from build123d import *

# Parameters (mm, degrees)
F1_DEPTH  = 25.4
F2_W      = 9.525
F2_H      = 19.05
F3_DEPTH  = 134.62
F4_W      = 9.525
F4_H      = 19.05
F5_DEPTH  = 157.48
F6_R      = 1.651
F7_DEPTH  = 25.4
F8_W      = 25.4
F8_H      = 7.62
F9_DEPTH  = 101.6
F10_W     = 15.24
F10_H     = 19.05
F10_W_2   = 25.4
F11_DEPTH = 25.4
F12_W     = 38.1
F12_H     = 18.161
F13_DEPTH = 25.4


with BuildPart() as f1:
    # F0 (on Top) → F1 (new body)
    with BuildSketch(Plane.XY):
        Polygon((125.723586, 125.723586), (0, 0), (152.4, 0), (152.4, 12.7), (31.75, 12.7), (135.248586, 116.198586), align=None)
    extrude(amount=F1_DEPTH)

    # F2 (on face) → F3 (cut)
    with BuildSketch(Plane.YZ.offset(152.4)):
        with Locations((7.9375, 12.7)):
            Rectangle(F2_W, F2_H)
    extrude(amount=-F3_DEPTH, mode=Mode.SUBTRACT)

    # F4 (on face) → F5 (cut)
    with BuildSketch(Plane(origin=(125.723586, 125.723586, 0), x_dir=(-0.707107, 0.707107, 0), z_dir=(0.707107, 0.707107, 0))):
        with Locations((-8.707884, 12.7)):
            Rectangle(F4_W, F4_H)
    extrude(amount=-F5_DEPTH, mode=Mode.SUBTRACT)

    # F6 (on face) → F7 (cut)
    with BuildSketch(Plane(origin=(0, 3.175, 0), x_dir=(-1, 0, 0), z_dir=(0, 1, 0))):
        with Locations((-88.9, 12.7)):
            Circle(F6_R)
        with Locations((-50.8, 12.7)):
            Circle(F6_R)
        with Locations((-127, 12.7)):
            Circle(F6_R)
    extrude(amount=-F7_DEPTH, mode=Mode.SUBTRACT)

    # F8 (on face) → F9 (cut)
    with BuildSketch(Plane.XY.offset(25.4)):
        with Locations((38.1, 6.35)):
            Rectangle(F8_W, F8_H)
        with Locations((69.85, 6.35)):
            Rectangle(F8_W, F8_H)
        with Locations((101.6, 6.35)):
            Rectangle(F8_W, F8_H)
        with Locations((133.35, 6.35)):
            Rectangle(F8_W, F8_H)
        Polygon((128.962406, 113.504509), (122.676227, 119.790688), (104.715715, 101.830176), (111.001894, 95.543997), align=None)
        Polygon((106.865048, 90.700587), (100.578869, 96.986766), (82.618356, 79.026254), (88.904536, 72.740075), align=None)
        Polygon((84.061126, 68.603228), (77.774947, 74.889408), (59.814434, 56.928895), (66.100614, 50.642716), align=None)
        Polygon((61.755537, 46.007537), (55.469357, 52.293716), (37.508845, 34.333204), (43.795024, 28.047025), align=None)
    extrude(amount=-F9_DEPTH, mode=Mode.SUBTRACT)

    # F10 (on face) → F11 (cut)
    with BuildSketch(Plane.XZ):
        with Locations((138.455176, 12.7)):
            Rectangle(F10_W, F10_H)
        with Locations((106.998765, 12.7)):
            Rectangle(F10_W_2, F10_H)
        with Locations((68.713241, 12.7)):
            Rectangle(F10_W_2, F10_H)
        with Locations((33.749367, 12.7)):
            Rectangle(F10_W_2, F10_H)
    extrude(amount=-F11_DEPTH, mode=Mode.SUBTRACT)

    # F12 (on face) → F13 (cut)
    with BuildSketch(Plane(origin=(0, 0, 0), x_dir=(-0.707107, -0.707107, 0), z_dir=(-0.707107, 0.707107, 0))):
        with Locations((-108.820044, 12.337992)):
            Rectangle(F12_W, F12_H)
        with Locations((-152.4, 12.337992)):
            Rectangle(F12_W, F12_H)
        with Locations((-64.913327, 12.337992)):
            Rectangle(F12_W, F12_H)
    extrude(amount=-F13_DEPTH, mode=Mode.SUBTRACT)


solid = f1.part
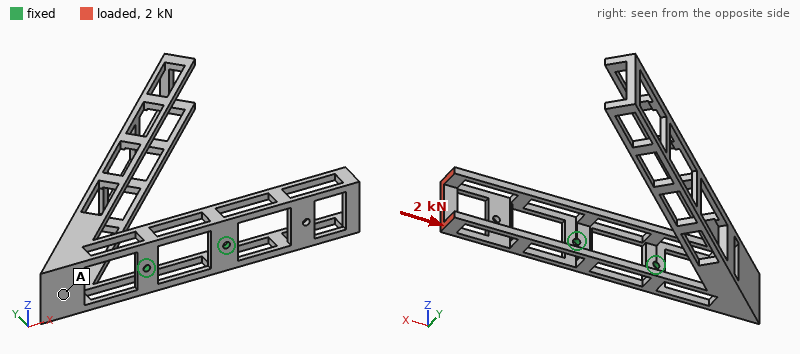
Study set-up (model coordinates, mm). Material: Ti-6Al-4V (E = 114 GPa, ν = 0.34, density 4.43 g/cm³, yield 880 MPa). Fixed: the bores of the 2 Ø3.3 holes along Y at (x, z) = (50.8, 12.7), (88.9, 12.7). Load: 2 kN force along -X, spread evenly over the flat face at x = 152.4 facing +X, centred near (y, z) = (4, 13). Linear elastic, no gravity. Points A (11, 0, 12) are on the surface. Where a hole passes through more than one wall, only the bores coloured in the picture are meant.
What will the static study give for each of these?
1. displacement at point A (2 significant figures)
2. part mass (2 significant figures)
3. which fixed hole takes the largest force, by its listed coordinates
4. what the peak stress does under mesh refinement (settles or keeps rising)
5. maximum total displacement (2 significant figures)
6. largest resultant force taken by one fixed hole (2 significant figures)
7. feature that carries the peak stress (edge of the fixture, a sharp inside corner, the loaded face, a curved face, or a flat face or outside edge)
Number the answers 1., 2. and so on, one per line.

1. 0.096 mm
2. 96 g
3. (88.9, 12.7)
4. keeps rising
5. 0.34 mm
6. 1.5 kN
7. edge of the fixture
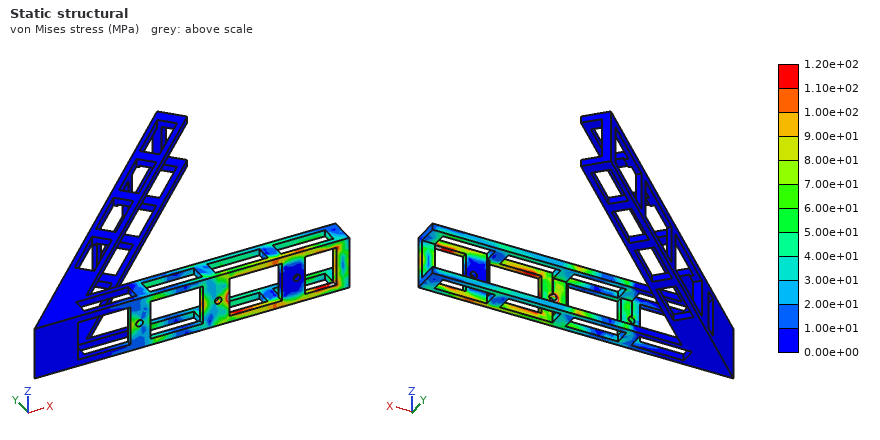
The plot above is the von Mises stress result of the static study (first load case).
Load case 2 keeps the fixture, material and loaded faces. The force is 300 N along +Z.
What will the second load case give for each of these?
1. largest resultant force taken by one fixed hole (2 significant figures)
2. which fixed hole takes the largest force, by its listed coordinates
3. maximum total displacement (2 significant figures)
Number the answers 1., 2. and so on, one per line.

1. 400 N
2. (88.9, 12.7)
3. 0.81 mm
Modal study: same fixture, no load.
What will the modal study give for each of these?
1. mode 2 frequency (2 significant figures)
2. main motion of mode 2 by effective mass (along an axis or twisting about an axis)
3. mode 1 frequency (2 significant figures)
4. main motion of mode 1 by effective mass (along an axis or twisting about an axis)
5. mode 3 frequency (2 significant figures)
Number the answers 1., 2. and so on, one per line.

1. 250 Hz
2. along X
3. 160 Hz
4. along Z
5. 650 Hz
